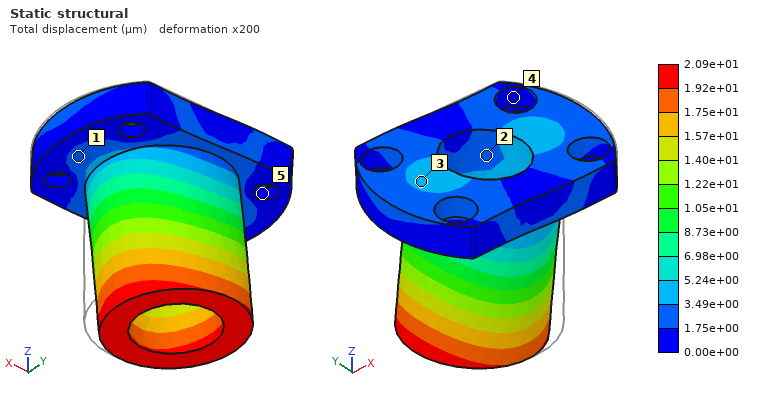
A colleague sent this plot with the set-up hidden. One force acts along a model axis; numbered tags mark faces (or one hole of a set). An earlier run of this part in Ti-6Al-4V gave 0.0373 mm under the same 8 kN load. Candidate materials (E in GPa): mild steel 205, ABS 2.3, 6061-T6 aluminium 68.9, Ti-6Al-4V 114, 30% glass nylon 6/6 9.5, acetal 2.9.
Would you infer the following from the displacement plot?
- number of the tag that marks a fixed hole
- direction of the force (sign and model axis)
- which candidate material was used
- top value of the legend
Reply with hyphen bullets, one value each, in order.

- 5
- -X
- mild steel
- 2.09e+01 µm
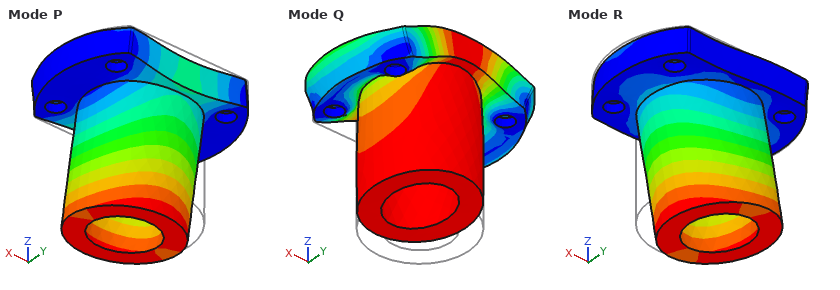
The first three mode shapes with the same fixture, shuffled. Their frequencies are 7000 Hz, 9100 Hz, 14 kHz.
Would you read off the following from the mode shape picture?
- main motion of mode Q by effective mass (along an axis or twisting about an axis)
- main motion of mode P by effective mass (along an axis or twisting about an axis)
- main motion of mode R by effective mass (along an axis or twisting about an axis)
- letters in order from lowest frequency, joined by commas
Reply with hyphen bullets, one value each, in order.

- along Z
- along Y
- along X
- P, R, Q
